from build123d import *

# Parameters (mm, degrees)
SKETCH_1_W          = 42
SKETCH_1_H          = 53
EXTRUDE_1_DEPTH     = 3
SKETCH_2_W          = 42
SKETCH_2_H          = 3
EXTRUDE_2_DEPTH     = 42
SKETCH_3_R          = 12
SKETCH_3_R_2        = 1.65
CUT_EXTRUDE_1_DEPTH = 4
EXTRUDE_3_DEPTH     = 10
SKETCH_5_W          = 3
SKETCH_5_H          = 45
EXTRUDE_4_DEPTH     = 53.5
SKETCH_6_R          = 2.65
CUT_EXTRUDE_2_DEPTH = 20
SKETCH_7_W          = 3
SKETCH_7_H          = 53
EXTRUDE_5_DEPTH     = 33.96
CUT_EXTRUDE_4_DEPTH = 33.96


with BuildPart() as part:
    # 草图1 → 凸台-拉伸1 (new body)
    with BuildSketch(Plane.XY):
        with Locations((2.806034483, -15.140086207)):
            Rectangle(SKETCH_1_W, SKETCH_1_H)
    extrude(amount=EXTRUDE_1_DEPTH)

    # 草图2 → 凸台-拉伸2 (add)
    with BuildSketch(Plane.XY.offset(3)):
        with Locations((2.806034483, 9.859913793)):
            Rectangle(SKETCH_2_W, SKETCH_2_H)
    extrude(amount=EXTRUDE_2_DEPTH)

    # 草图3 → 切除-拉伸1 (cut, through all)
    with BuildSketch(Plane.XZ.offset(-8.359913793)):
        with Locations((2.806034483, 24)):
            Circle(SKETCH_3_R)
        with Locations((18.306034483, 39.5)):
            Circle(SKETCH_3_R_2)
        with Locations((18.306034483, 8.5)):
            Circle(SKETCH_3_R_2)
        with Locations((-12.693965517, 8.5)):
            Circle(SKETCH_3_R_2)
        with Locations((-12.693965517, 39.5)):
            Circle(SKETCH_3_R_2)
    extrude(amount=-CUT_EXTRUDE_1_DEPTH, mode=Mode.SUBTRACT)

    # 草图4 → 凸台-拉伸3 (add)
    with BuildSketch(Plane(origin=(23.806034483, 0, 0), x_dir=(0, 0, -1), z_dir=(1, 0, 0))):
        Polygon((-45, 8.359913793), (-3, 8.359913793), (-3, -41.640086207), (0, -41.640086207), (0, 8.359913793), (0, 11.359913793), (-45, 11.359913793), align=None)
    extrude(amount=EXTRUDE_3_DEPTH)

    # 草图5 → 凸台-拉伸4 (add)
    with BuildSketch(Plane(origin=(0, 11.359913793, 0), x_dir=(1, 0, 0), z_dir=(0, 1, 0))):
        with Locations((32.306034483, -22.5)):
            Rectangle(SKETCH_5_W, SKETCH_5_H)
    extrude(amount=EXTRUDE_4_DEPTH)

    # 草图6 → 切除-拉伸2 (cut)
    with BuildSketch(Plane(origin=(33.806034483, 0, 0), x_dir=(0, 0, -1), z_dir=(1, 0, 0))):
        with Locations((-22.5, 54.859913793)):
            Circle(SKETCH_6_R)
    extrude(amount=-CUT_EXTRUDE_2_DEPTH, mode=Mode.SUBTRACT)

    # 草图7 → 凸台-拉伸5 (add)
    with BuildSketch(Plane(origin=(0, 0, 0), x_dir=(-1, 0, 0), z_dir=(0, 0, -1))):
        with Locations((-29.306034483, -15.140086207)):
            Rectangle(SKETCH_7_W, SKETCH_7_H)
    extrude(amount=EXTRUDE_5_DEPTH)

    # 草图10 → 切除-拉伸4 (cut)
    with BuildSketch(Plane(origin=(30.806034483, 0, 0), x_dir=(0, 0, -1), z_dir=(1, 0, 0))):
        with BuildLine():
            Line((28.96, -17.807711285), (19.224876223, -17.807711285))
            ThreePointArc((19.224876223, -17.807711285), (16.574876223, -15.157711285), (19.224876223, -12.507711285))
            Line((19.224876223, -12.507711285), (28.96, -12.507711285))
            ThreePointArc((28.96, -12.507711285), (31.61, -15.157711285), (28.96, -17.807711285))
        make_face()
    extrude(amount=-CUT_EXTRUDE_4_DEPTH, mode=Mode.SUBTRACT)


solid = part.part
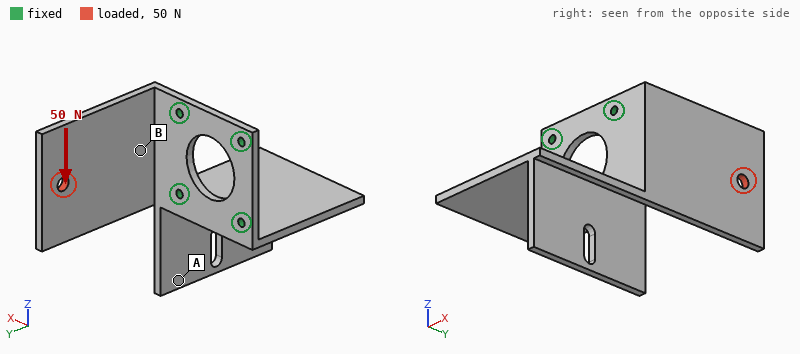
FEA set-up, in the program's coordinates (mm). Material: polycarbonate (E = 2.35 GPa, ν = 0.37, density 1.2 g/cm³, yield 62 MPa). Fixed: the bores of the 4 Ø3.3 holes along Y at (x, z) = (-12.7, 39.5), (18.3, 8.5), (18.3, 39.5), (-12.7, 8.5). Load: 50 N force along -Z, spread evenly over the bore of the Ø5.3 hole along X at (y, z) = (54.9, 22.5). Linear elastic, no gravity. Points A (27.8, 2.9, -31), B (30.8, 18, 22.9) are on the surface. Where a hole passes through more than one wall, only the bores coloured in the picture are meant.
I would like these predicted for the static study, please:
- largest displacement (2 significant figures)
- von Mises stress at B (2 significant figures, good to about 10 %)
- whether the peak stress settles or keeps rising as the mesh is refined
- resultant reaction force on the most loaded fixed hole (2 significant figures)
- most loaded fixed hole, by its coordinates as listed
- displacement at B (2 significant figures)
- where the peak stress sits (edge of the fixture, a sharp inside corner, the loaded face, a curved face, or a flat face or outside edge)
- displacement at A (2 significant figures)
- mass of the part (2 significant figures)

1.5 mm
3.2 MPa
keeps rising
87 N
(18.3, 8.5)
0.23 mm
edge of the fixture
0.47 mm
31 g
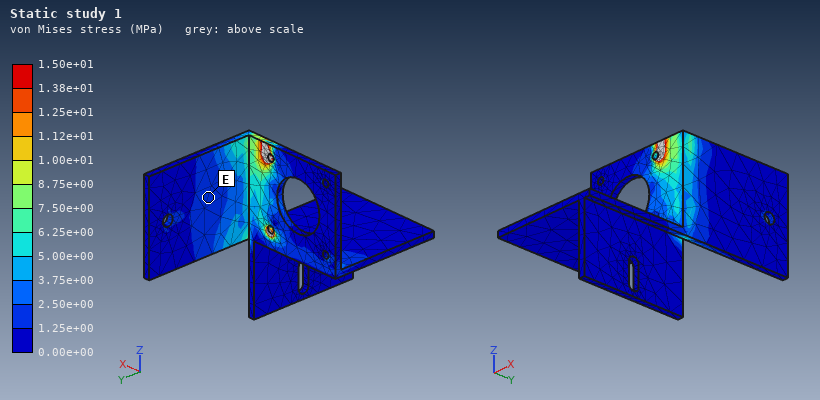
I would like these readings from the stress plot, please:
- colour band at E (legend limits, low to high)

1.25e+00 to 2.50e+00 MPa
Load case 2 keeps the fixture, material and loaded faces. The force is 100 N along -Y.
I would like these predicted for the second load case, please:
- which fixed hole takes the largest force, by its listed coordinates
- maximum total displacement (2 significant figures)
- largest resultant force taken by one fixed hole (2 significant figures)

(18.3, 8.5)
1.5 mm
73 N
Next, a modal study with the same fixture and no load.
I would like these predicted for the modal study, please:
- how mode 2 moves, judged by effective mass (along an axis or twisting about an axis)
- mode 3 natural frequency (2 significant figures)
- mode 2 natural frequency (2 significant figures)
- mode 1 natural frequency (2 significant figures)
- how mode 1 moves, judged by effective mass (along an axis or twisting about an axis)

along Z
350 Hz
210 Hz
190 Hz
along X
